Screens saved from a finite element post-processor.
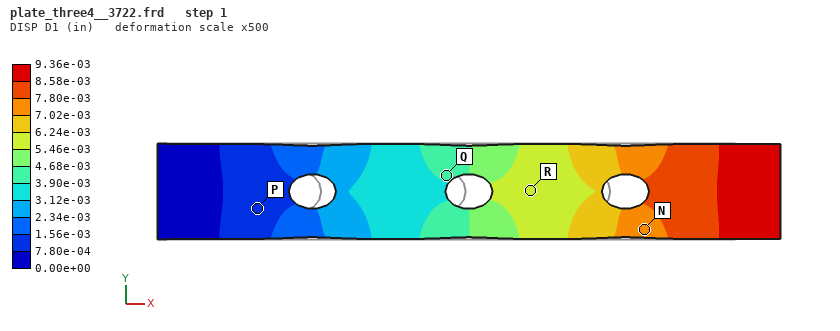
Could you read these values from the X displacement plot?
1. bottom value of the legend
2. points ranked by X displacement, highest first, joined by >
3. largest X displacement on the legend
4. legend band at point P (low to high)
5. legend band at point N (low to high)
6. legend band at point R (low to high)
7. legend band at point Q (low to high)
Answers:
0.00e+00 in
N > R > Q > P
9.36e-03 in
7.80e-04 to 1.56e-03 in
7.02e-03 to 7.80e-03 in
5.46e-03 to 6.24e-03 in
3.90e-03 to 4.68e-03 in
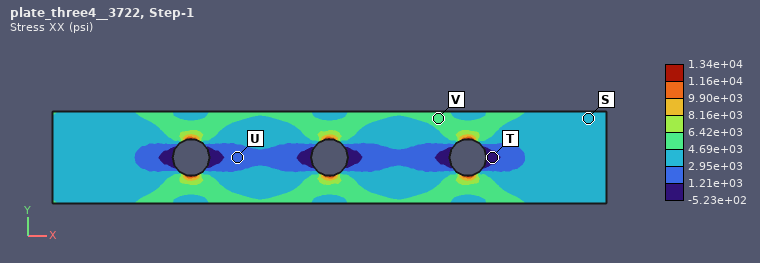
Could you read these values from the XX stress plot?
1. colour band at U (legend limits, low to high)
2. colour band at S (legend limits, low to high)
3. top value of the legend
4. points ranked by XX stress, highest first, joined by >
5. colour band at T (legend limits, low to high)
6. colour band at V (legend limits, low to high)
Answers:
1.21e+03 to 2.95e+03 psi
2.95e+03 to 4.69e+03 psi
1.34e+04 psi
V > S > U > T
-5.23e+02 to 1.21e+03 psi
4.69e+03 to 6.42e+03 psi
